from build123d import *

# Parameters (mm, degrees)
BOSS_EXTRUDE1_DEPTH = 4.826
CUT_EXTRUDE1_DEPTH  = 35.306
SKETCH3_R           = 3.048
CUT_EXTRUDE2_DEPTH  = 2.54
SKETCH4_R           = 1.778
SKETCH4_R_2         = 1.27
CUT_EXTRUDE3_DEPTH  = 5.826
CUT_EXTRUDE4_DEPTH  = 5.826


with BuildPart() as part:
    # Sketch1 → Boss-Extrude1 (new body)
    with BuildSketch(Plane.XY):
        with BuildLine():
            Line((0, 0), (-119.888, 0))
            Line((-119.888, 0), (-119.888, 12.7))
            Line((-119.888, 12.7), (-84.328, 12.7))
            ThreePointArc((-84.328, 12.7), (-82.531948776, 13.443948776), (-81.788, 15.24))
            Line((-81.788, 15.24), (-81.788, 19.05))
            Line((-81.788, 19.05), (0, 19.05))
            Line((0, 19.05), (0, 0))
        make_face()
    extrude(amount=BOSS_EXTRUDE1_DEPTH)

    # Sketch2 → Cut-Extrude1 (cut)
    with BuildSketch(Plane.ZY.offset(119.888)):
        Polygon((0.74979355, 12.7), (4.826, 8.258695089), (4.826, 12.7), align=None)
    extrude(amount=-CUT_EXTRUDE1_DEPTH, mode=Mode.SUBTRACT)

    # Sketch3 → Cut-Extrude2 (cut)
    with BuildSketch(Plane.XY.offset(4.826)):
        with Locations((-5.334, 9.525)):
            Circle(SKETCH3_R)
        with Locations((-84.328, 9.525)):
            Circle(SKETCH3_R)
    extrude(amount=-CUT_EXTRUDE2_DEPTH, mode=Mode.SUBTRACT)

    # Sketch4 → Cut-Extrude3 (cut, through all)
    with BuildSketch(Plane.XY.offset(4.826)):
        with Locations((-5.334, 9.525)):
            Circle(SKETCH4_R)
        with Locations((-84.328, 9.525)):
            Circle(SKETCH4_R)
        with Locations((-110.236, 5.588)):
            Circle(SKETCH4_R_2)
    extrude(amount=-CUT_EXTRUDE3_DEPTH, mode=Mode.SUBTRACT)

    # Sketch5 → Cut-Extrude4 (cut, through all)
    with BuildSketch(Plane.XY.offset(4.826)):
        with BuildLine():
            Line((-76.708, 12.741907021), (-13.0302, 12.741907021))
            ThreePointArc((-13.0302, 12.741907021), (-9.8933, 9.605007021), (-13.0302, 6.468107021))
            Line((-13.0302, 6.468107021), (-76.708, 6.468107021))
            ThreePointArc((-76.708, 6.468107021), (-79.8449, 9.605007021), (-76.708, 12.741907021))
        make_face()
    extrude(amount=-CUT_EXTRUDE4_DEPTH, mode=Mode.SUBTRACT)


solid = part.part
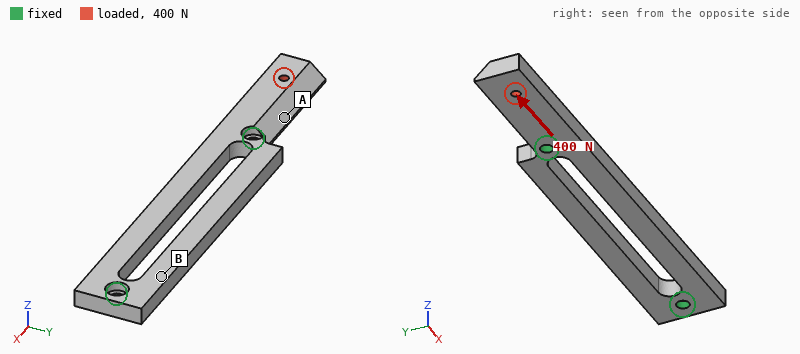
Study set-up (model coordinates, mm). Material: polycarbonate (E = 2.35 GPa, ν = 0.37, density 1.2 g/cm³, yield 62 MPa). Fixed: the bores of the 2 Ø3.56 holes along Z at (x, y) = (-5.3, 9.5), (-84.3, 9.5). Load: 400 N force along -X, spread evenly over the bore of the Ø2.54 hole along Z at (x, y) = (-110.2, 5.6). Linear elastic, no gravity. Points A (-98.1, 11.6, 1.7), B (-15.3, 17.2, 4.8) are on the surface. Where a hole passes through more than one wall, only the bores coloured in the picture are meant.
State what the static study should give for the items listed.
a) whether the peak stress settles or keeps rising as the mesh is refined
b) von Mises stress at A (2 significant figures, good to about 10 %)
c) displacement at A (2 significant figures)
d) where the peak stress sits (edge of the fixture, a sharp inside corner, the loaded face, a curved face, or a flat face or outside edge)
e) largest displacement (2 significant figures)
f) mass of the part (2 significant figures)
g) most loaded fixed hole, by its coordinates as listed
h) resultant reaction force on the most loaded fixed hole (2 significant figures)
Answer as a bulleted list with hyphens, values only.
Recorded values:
- keeps rising
- 8.1 MPa
- 0.25 mm
- edge of the fixture
- 0.82 mm
- 8.7 g
- (-84.3, 9.5)
- 330 N
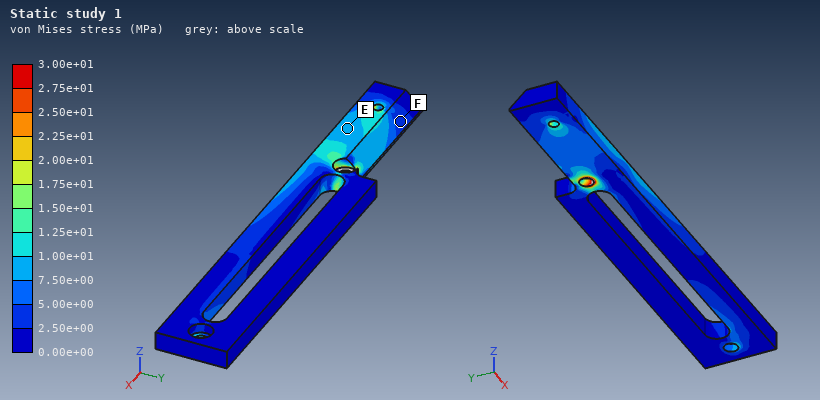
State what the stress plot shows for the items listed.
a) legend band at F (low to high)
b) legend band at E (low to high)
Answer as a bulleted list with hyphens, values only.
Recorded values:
- 2.50e+00 to 5.00e+00 MPa
- 7.50e+00 to 1.00e+01 MPa
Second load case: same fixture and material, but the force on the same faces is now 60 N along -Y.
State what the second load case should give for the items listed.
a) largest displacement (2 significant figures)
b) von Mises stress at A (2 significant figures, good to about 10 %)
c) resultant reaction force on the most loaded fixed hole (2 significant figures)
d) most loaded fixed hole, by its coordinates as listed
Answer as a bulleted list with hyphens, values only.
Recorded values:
- 1.1 mm
- 7.8 MPa
- 81 N
- (-84.3, 9.5)
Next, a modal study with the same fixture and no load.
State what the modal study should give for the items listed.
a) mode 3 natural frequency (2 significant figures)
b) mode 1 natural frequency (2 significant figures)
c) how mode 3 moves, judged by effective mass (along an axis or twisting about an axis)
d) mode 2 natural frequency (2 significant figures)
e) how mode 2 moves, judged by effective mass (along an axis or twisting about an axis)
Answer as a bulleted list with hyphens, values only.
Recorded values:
- 970 Hz
- 600 Hz
- along Z
- 850 Hz
- along Z
